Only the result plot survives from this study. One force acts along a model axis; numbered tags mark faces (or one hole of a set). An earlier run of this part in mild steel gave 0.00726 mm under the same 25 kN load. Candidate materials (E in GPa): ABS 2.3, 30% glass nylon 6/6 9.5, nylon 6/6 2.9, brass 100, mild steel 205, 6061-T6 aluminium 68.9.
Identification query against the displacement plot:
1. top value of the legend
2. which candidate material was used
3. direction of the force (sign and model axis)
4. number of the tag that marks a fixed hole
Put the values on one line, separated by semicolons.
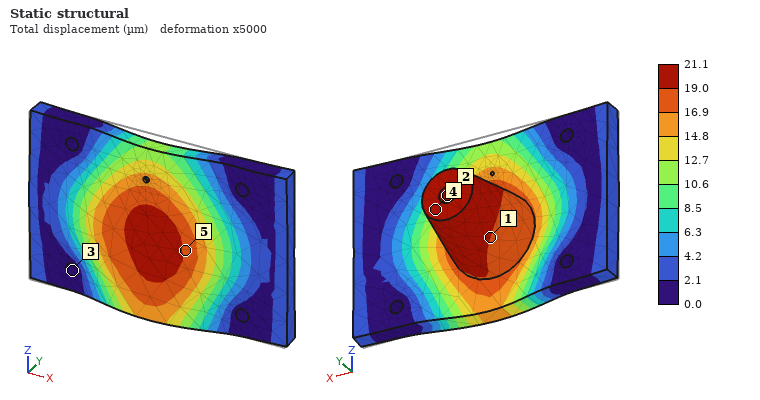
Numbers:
21.1 µm; 6061-T6 aluminium; -Y; 3
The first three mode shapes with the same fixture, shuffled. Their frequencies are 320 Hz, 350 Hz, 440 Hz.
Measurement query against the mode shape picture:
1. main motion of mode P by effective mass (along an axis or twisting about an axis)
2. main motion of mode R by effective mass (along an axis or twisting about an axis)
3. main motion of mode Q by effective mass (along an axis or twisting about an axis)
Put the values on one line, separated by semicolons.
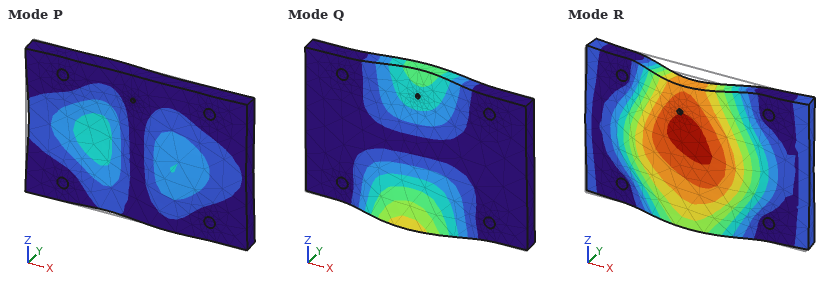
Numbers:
along X; along Y; along Z
